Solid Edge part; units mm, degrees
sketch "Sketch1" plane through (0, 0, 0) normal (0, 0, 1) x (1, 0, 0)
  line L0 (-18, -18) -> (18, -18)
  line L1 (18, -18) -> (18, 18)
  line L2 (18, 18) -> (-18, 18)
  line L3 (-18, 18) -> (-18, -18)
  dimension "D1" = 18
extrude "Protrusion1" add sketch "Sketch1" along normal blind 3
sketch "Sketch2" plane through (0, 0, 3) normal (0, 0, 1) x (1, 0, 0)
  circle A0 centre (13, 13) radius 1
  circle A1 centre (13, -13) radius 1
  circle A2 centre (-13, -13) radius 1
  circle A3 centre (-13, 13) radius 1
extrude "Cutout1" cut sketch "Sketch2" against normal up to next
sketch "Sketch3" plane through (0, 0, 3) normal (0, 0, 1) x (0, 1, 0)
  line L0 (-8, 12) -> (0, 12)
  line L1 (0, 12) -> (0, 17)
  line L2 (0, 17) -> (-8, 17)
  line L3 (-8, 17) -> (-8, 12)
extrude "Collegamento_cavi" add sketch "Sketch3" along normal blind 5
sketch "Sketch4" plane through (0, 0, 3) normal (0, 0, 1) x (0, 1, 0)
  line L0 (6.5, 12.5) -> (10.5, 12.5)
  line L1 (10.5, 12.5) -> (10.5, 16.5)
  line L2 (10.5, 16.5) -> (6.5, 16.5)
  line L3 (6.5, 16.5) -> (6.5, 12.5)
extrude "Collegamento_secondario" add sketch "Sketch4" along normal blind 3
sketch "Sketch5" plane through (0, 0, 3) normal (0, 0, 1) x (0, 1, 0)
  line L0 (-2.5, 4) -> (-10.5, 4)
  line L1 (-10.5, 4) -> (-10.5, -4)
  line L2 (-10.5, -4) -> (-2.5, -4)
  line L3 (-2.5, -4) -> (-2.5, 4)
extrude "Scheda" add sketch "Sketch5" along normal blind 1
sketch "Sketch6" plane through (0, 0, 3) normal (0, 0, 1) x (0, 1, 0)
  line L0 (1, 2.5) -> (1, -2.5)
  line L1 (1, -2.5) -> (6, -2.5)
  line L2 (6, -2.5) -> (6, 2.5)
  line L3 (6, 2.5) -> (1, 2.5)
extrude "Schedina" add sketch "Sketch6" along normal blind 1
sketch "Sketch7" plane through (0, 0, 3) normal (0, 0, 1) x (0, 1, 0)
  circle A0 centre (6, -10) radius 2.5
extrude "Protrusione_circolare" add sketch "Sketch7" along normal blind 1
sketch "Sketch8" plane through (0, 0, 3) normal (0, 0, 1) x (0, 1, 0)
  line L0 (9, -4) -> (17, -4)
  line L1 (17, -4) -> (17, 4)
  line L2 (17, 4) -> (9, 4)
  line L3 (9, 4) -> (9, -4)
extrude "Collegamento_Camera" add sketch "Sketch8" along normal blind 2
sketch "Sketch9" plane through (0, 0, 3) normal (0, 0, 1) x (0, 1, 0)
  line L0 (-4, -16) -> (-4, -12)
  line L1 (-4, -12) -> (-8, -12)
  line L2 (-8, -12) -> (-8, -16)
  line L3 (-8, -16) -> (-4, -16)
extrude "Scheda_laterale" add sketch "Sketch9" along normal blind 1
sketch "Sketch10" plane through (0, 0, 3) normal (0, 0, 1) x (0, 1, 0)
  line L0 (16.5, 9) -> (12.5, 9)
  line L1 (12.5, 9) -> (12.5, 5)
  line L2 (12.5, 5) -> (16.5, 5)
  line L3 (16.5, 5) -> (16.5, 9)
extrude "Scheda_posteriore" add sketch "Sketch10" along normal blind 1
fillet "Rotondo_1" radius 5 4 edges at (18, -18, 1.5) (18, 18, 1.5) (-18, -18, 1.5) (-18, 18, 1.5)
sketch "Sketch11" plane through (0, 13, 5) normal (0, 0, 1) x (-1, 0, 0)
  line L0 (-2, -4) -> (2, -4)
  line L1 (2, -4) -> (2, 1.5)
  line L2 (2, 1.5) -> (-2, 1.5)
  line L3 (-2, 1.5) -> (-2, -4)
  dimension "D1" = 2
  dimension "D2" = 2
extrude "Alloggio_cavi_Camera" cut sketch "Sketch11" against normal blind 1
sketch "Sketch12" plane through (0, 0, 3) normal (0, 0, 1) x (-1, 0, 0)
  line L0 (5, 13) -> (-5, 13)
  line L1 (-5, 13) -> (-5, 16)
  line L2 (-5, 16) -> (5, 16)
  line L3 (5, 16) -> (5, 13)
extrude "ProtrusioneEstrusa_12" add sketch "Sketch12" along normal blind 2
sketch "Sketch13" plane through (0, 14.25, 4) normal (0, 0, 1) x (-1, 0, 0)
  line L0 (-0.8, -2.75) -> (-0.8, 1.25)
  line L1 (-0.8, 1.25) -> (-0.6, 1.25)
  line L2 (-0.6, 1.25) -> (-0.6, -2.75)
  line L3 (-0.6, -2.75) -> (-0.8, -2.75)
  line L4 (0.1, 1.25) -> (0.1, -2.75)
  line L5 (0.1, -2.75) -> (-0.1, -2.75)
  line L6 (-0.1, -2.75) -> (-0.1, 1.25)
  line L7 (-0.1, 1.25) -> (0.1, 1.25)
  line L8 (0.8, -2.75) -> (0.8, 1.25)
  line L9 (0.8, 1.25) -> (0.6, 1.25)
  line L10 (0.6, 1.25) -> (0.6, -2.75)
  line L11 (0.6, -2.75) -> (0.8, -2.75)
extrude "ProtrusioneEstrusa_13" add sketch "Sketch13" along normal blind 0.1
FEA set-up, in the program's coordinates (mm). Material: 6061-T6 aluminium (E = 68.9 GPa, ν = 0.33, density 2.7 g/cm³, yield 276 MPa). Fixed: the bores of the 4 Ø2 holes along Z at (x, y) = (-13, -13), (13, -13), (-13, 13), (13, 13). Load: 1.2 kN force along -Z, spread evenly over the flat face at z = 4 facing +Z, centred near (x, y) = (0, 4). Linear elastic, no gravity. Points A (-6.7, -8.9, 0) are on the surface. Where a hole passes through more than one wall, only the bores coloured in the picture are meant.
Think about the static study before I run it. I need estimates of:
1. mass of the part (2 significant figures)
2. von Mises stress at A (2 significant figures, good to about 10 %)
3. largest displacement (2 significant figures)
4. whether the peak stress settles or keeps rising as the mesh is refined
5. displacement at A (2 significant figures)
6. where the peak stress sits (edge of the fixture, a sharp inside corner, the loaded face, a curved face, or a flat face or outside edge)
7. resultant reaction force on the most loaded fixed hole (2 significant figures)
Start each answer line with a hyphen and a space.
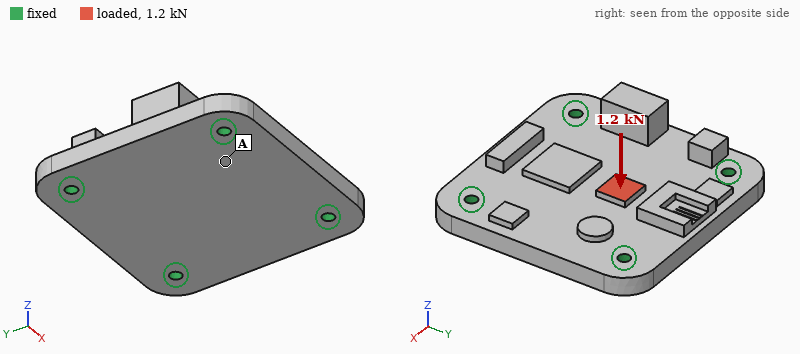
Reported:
- 12 g
- 27 MPa
- 56 µm
- keeps rising
- 18 µm
- edge of the fixture
- 410 N
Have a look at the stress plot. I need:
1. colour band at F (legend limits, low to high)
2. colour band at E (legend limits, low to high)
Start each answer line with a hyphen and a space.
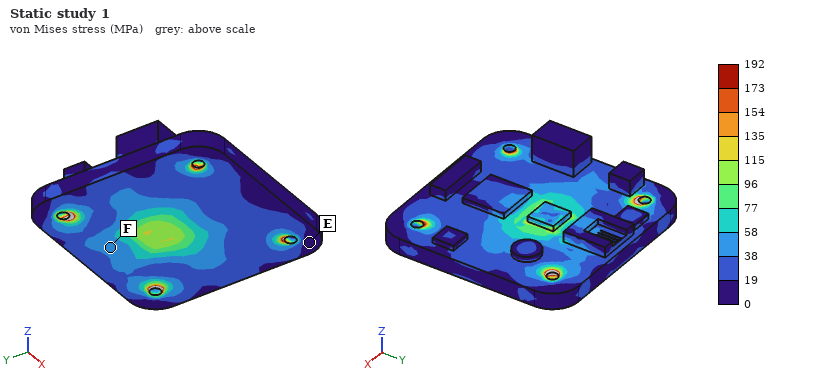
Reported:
- 38 to 58 MPa
- 0 to 19 MPa
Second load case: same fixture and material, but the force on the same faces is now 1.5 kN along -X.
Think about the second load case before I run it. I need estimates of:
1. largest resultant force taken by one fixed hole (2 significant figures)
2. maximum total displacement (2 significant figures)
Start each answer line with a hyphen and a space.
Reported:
- 510 N
- 17 µm
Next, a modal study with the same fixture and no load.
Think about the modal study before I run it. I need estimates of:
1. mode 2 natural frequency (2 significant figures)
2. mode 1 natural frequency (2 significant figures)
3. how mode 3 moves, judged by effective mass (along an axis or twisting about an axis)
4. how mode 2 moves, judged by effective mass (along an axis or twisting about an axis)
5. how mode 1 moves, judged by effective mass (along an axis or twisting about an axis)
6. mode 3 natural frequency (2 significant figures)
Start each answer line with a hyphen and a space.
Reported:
- 19 kHz
- 15 kHz
- twisting about X
- twisting about Y
- along Z
- 22 kHz
